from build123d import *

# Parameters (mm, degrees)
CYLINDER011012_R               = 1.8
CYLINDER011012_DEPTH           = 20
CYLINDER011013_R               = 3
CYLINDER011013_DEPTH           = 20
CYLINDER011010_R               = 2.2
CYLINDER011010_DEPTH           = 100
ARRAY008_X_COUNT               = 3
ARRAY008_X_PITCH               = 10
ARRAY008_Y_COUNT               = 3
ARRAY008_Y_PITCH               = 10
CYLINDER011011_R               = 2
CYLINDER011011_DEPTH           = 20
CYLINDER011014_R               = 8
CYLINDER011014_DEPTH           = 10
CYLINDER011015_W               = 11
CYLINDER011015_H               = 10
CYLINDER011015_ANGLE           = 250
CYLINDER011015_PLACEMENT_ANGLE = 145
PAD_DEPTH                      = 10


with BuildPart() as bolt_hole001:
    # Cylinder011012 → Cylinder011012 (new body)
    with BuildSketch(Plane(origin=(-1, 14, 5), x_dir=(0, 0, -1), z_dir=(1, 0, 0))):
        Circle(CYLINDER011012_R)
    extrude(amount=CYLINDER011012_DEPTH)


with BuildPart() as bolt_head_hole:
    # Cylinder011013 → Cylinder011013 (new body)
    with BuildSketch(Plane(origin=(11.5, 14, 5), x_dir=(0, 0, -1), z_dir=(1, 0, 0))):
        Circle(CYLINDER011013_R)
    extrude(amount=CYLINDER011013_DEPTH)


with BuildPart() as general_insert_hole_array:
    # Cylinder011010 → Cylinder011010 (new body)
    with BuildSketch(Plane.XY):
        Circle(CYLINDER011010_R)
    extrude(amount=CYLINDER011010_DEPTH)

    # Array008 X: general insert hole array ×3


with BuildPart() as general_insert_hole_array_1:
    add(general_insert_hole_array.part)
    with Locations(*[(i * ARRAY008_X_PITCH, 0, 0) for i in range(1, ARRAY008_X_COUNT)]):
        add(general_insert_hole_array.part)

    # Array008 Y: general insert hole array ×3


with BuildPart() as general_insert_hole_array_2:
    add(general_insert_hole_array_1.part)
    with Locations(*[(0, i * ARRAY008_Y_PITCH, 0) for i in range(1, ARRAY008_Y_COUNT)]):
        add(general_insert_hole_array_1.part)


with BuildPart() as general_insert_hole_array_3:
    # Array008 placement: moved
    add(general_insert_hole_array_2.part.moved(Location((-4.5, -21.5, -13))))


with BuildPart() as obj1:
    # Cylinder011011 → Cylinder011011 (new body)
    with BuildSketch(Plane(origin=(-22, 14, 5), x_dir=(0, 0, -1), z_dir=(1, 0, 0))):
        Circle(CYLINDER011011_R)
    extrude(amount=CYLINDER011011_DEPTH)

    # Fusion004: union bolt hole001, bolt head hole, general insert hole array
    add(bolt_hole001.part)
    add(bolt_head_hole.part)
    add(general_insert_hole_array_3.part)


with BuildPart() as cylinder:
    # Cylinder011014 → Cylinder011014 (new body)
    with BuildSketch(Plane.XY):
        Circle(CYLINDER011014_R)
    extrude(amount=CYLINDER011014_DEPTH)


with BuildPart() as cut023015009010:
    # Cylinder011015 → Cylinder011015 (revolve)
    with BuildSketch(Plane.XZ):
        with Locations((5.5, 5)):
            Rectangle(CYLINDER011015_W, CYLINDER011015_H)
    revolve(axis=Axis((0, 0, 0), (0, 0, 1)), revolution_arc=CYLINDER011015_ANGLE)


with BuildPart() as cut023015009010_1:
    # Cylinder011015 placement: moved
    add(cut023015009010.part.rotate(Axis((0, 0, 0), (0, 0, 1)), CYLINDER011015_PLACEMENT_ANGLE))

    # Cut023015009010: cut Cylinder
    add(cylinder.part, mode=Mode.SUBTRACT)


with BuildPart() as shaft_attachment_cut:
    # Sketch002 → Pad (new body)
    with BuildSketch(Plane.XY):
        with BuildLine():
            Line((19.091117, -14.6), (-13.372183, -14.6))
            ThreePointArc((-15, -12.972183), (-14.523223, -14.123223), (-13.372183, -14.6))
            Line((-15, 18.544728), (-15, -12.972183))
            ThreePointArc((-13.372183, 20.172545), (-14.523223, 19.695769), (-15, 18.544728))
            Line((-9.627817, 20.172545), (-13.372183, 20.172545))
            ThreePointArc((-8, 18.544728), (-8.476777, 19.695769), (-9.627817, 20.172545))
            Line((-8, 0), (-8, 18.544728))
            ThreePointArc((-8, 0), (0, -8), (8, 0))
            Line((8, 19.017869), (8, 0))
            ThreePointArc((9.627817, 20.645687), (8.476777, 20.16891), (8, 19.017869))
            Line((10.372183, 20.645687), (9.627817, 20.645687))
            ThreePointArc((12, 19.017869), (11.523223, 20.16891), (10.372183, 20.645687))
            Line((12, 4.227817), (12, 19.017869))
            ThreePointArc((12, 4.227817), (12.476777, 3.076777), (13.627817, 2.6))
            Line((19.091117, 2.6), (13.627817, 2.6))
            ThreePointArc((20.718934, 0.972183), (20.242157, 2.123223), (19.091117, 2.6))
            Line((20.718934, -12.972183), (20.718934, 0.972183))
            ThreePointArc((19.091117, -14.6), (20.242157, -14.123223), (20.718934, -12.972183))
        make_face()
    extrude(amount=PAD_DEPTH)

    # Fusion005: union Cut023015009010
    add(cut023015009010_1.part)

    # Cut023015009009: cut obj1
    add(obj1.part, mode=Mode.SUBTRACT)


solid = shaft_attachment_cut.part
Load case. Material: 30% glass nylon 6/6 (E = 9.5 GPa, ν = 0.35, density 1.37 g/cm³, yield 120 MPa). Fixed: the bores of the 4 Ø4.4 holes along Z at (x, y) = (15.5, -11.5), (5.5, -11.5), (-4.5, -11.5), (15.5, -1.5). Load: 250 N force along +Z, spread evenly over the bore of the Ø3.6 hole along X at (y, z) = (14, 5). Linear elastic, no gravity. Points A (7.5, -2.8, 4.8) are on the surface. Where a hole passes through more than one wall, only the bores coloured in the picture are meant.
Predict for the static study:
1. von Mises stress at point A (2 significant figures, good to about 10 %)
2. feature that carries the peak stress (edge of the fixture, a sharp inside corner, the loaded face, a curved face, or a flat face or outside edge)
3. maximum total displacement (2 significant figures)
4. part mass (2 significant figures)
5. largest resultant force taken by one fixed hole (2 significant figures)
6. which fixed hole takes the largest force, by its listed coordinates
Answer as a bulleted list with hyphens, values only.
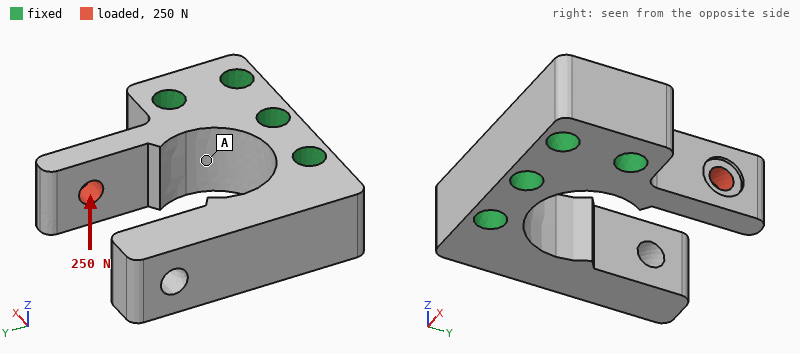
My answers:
- 5.1 MPa
- a curved face
- 0.20 mm
- 8.2 g
- 340 N
- (15.5, -1.5)
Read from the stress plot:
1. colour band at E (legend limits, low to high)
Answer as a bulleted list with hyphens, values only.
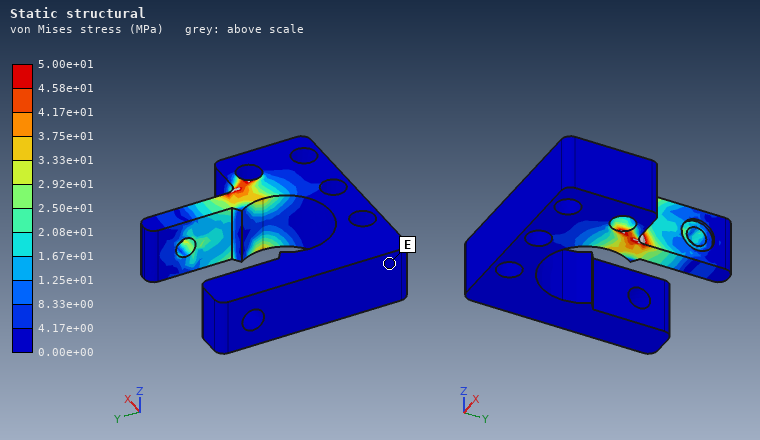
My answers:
- 0.00e+00 to 4.17e+00 MPa
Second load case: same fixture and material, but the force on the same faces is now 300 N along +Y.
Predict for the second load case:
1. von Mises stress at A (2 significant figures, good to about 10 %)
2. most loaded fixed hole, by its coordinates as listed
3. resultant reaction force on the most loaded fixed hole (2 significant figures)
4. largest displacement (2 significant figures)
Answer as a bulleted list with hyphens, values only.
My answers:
- 7.2 MPa
- (15.5, -1.5)
- 140 N
- 44 µm
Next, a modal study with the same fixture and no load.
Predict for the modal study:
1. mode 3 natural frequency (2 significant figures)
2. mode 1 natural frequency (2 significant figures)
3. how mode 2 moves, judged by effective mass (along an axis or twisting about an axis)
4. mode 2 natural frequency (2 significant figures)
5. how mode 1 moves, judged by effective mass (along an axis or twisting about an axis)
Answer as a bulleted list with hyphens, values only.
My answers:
- 4900 Hz
- 3300 Hz
- along Z
- 4000 Hz
- along X
